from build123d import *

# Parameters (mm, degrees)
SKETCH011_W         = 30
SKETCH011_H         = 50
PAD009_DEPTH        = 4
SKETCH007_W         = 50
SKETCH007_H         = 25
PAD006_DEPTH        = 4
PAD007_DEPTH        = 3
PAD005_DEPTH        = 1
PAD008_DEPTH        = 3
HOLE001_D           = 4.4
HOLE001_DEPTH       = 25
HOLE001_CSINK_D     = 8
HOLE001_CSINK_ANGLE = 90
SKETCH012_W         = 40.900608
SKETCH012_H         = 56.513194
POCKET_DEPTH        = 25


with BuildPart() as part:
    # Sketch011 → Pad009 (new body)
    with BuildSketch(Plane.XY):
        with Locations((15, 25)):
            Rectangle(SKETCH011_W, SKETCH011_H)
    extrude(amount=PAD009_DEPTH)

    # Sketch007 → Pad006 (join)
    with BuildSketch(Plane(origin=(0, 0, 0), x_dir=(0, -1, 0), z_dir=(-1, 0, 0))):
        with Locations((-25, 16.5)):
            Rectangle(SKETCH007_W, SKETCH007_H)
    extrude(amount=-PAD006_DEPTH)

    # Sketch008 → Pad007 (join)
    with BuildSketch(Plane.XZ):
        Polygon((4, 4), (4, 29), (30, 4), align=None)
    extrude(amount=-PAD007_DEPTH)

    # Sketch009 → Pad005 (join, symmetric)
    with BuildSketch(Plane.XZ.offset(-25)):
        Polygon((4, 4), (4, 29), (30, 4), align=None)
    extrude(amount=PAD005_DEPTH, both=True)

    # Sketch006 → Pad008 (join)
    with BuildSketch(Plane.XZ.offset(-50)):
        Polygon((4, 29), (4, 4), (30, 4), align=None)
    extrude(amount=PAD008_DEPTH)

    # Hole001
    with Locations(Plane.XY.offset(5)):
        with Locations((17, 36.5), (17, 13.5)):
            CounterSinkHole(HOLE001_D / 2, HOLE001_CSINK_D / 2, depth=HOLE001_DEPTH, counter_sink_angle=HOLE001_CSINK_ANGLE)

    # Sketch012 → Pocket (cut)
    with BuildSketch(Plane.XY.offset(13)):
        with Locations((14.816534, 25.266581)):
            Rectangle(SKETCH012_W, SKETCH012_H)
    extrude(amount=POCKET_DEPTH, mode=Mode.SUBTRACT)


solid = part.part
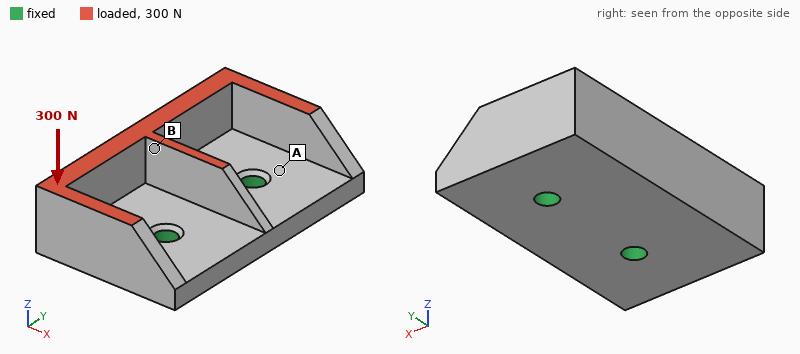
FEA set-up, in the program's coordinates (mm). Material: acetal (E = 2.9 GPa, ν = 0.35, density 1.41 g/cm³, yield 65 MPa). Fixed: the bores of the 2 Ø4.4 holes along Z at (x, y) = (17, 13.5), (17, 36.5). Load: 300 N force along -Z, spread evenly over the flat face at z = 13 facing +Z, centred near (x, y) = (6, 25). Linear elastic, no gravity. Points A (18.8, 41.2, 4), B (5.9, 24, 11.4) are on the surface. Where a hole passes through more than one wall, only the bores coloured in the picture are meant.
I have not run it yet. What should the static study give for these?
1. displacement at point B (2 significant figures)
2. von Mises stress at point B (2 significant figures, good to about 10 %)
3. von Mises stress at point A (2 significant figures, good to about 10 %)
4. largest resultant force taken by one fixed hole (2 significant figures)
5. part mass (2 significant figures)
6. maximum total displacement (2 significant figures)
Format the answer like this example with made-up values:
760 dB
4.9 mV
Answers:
0.27 mm
4.7 MPa
8.8 MPa
150 N
13 g
0.40 mm
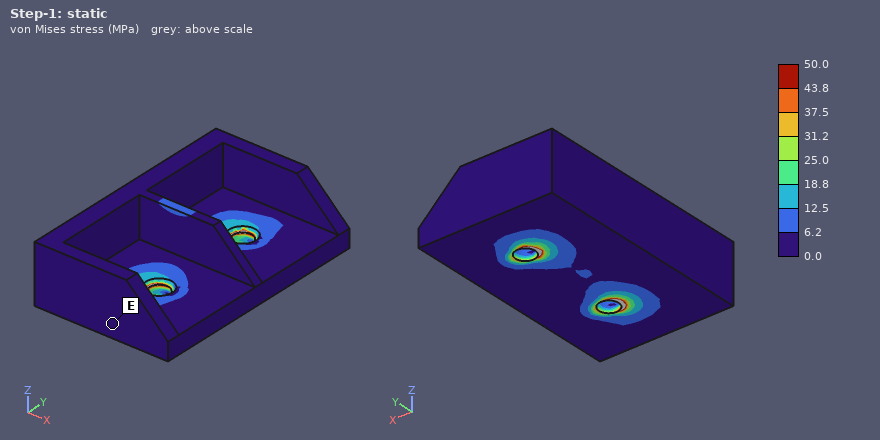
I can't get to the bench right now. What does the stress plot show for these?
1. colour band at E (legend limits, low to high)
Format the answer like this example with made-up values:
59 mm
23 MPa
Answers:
0.0 to 6.2 MPa
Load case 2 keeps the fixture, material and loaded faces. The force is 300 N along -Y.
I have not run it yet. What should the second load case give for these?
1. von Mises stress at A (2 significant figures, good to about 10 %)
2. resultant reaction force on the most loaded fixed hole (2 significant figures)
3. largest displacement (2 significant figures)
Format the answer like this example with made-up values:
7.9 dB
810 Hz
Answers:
10.0 MPa
230 N
0.39 mm
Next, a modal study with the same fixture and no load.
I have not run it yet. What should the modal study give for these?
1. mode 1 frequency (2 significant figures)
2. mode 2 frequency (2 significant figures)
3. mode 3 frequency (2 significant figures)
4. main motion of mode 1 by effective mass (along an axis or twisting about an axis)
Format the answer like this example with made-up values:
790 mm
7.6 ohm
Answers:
1700 Hz
2000 Hz
3300 Hz
along Z
